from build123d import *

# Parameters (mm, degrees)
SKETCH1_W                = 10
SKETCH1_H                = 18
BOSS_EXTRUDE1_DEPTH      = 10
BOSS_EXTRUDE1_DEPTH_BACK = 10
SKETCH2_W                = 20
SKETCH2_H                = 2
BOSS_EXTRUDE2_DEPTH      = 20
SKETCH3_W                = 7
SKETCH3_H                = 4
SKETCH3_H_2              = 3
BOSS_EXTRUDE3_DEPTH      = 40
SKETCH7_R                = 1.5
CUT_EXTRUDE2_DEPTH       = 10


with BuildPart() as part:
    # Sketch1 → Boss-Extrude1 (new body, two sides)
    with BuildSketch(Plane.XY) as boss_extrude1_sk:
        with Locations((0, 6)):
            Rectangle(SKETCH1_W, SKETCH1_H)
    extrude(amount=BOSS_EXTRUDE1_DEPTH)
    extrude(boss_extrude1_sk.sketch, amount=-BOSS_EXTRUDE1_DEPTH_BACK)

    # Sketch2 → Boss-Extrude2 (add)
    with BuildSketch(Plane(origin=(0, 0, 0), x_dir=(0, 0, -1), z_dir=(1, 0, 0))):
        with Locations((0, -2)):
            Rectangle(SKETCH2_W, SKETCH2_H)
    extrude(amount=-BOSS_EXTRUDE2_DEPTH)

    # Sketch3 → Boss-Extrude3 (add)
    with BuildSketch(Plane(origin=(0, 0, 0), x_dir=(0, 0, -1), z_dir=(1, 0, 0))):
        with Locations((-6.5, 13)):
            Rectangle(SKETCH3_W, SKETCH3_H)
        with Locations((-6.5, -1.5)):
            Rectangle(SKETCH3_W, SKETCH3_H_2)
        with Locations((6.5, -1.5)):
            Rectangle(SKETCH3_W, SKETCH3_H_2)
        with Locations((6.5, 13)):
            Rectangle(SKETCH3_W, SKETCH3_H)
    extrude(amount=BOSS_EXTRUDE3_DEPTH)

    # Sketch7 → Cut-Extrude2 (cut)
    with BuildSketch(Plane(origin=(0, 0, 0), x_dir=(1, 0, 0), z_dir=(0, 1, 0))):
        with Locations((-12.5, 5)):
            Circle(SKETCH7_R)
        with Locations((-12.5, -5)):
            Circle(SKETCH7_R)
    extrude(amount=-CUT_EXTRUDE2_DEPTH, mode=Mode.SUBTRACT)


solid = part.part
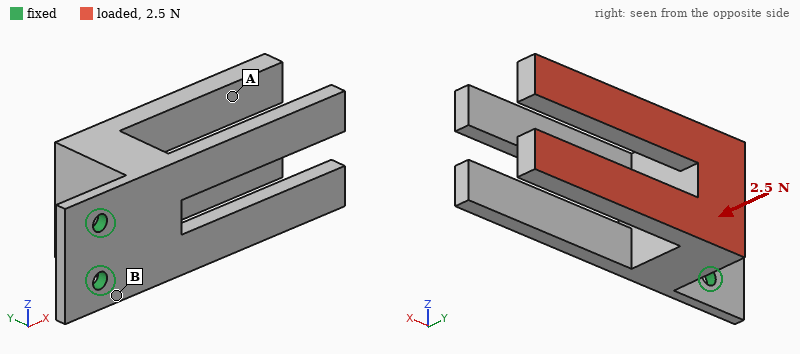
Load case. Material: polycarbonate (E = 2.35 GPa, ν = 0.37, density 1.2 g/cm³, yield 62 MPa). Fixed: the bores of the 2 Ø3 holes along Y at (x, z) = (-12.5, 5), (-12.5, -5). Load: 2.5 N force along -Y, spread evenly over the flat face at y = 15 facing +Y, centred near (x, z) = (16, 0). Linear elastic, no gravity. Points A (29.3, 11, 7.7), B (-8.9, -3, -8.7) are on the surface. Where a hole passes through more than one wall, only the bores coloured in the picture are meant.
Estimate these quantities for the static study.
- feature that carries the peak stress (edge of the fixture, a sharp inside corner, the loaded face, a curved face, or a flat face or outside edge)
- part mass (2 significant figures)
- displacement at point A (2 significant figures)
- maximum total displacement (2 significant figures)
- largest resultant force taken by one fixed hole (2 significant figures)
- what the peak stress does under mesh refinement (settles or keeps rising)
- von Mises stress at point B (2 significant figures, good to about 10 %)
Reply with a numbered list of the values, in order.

1. edge of the fixture
2. 9.1 g
3. 0.58 mm
4. 0.77 mm
5. 1.3 N
6. keeps rising
7. 4.1 MPa
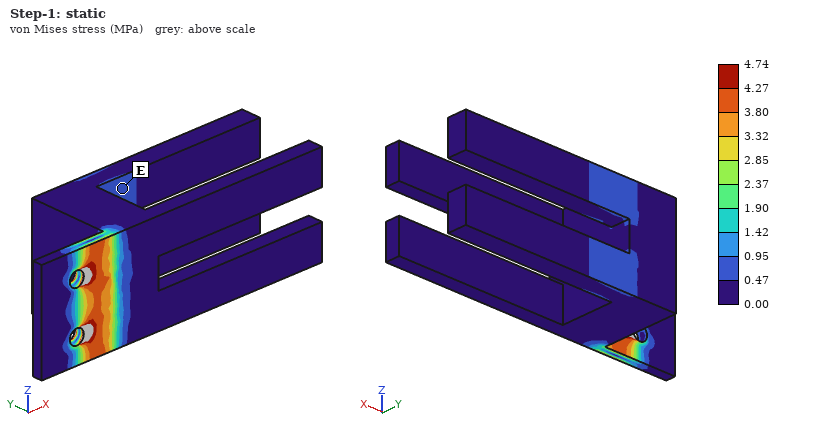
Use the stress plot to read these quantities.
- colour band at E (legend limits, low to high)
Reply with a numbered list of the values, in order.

1. 0.47 to 0.95 MPa
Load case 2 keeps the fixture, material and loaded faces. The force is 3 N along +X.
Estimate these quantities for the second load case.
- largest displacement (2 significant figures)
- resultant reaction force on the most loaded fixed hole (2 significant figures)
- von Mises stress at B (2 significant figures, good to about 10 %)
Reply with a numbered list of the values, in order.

1. 0.61 mm
2. 1.6 N
3. 3.3 MPa
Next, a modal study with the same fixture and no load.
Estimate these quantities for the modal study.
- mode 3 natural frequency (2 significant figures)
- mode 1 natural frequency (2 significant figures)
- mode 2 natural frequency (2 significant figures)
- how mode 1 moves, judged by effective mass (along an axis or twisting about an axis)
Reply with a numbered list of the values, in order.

1. 550 Hz
2. 140 Hz
3. 500 Hz
4. along Y
